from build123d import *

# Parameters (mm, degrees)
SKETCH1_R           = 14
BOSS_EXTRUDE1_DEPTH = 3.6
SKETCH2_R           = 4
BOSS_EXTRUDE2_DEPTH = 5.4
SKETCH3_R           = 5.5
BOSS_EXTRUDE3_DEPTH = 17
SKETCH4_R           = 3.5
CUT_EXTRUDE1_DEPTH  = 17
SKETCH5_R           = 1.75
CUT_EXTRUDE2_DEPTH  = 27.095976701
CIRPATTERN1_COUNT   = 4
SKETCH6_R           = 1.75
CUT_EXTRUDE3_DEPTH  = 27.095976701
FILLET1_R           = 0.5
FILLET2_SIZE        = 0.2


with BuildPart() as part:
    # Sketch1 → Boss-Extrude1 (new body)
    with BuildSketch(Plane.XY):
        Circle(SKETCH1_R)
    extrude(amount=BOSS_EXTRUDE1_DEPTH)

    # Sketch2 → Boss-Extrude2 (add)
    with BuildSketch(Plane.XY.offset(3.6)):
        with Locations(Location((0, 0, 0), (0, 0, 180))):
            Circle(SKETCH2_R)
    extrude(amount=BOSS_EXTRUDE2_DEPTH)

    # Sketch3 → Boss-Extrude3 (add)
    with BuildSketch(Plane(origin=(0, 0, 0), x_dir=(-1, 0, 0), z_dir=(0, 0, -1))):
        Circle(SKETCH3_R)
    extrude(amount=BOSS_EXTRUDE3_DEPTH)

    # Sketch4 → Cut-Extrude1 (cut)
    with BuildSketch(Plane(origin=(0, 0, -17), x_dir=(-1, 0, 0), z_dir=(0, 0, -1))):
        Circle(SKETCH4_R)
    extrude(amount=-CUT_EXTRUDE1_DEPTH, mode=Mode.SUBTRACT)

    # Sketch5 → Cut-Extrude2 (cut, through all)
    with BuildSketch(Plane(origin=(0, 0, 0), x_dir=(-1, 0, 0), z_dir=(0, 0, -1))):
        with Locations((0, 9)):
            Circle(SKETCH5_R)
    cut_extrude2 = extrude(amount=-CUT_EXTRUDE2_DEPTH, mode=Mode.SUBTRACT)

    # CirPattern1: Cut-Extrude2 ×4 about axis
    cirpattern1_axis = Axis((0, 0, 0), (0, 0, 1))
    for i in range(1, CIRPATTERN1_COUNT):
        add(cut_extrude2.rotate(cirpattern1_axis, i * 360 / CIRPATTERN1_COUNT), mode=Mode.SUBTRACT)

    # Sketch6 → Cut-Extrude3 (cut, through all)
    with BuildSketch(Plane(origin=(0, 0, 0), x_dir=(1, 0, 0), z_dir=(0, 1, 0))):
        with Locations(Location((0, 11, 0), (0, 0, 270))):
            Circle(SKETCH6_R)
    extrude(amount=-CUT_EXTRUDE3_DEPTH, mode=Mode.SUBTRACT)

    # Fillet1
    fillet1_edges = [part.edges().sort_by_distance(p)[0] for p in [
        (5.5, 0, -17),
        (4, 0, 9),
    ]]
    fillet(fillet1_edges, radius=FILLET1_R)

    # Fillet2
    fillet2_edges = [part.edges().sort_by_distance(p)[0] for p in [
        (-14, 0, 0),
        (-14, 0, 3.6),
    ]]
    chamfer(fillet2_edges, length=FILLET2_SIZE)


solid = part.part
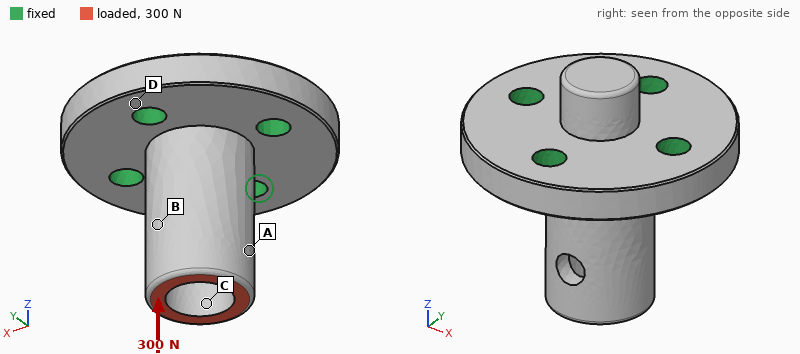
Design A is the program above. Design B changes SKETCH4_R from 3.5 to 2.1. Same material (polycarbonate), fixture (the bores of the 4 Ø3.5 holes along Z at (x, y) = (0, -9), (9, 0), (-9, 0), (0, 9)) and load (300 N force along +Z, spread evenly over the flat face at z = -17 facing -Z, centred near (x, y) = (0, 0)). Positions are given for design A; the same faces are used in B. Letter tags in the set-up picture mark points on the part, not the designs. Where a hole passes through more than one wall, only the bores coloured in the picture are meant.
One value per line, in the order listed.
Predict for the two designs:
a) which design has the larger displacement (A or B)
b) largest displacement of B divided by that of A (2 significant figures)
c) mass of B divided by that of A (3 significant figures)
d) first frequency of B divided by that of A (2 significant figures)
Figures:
A
0.77
1.12
0.93
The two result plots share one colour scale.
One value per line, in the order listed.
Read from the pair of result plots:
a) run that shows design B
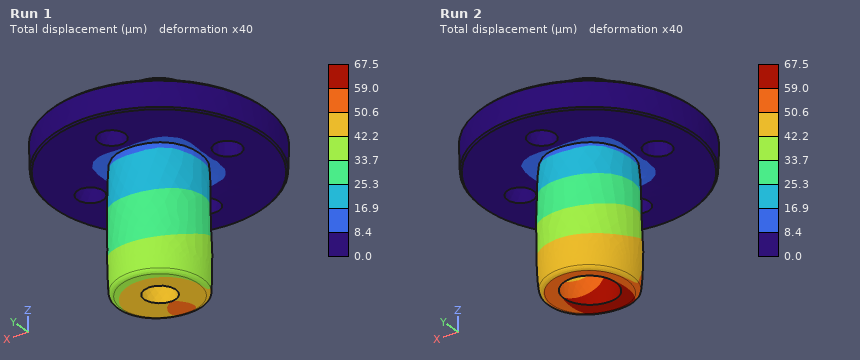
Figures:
Run 1
